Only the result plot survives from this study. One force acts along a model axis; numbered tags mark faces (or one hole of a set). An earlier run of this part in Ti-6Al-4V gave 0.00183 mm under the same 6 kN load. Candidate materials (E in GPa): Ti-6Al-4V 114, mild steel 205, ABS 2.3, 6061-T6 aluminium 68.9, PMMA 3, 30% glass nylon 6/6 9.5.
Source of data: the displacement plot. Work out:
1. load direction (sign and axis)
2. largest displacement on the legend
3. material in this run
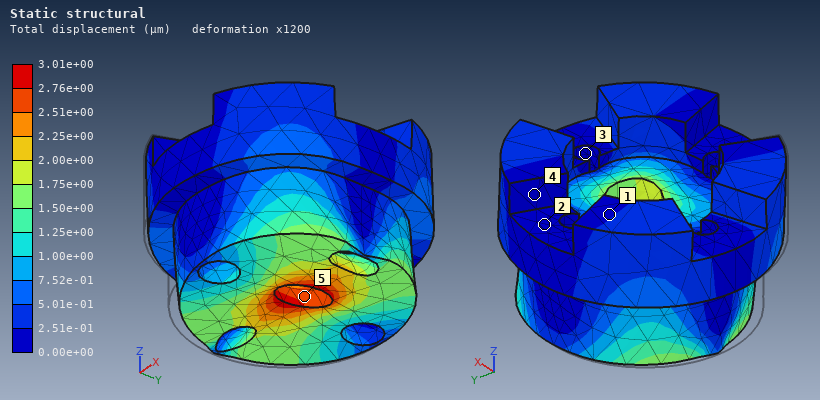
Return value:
+X
3.01e+00 µm
6061-T6 aluminium
